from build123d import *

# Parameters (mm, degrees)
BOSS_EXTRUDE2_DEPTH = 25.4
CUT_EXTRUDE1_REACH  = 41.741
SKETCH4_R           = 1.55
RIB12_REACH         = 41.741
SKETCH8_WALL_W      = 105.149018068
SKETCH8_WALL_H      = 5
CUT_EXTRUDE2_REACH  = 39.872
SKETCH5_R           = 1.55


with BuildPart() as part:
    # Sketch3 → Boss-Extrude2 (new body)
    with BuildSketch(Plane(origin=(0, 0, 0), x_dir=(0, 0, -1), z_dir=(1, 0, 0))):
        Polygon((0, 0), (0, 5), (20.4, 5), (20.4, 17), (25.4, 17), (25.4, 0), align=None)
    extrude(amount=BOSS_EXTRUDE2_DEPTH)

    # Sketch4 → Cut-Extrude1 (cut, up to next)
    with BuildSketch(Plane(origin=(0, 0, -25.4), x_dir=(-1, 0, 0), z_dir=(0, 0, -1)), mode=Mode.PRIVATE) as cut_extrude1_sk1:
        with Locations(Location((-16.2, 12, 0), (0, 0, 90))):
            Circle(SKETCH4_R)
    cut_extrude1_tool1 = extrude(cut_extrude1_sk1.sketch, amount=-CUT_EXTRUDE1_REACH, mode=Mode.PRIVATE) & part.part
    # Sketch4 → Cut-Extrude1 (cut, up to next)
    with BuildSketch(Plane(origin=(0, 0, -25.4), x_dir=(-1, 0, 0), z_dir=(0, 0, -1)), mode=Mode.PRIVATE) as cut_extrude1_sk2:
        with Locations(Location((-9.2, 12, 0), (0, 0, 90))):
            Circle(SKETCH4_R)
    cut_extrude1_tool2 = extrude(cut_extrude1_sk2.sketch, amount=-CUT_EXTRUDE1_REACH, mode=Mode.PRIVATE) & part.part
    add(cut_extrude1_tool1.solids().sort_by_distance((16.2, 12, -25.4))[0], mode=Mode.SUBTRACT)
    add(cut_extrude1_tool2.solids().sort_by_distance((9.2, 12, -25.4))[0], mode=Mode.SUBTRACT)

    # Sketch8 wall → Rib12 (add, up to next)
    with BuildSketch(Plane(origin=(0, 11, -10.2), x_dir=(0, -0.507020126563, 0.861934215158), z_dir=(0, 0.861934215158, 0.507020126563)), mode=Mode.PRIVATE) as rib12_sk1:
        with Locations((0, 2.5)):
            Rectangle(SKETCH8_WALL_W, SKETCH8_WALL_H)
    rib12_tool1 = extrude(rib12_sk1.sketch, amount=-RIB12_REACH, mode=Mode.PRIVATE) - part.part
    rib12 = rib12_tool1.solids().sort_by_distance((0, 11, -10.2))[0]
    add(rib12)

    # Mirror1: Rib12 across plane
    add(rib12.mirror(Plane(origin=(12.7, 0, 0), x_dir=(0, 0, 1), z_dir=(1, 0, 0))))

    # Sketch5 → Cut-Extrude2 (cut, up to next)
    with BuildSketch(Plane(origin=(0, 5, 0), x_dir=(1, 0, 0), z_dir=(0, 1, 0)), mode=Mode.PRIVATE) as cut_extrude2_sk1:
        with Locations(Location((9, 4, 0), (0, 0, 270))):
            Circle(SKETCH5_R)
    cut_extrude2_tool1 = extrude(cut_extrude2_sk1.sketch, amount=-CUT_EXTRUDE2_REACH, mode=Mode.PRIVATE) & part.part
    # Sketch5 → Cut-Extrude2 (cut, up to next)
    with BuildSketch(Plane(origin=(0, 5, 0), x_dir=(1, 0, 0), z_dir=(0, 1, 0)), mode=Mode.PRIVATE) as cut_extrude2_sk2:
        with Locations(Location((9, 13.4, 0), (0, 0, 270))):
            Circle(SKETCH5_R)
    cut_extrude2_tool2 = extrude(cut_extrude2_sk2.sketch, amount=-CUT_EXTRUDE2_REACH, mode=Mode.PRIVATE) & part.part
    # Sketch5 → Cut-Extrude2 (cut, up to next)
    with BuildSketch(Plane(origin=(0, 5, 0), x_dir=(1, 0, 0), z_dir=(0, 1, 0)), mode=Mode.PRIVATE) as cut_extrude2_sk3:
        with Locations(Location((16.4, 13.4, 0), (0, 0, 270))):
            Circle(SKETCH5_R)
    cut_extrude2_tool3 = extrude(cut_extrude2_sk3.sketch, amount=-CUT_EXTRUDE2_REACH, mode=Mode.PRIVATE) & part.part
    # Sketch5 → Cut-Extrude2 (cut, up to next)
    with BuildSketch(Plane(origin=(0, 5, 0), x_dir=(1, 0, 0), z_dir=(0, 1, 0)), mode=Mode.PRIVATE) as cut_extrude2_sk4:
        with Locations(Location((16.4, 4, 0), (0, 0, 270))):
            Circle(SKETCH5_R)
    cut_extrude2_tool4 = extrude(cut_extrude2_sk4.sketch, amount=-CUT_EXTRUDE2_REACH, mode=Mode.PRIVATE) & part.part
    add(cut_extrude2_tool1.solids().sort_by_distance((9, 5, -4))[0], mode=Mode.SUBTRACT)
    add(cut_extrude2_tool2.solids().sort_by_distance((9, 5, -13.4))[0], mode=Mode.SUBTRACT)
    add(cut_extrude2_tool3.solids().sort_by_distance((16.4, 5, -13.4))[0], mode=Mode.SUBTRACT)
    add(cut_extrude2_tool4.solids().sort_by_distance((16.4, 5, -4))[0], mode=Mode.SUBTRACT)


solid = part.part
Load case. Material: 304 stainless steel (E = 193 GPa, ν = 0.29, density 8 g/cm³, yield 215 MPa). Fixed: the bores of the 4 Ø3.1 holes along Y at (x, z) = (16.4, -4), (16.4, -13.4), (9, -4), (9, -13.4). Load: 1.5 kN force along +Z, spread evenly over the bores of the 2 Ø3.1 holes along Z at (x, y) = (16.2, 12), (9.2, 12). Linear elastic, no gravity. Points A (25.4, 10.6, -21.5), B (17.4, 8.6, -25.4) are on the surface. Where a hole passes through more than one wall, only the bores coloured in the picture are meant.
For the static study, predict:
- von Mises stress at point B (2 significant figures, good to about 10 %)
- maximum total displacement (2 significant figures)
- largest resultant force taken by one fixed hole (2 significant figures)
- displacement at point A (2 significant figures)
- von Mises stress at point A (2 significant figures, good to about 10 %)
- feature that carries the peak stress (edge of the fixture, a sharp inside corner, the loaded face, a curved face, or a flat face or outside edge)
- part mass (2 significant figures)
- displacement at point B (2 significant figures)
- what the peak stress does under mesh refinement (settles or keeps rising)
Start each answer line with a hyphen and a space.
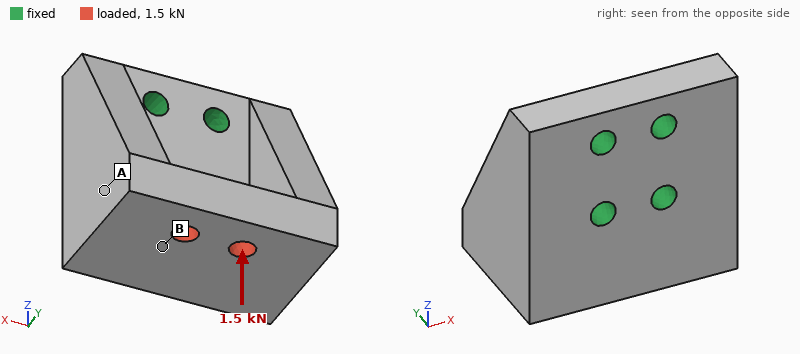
- 39 MPa
- 14 µm
- 740 N
- 5.1 µm
- 20 MPa
- edge of the fixture
- 46 g
- 8.4 µm
- keeps rising
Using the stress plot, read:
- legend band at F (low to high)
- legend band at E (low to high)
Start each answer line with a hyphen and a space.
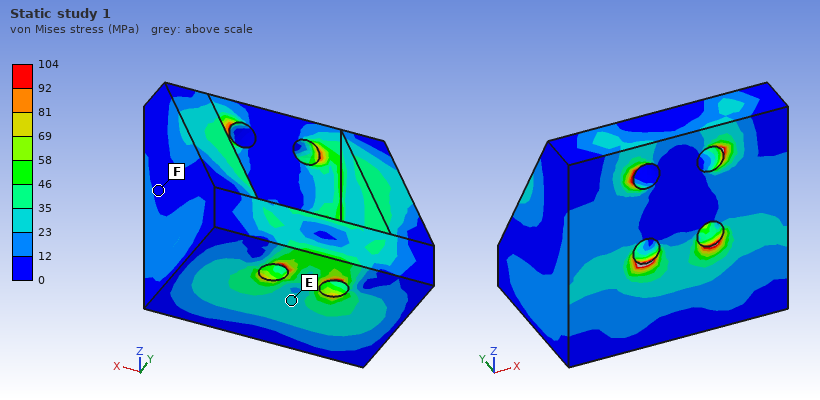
- 0 to 12 MPa
- 23 to 35 MPa
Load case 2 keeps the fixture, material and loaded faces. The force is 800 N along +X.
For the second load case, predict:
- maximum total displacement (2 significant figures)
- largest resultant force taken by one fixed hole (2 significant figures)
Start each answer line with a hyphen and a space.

- 8.3 µm
- 760 N
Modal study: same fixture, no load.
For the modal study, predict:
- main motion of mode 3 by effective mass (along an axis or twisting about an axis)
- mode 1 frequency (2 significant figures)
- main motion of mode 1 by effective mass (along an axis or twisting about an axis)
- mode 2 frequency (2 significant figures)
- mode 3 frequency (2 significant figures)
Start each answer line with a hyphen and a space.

- along X
- 13 kHz
- along X
- 14 kHz
- 25 kHz
